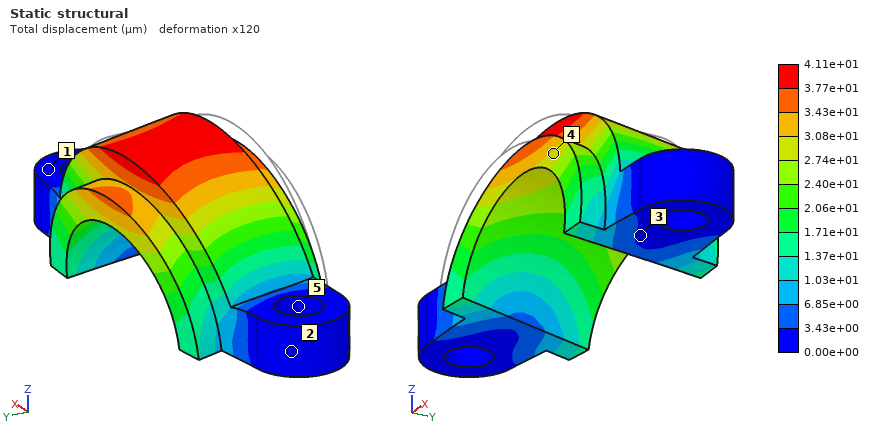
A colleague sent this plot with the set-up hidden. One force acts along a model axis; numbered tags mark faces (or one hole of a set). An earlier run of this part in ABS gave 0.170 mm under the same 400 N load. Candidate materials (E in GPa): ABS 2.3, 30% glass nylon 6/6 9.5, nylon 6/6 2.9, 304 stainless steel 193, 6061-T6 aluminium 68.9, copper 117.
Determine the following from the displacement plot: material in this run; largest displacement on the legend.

30% glass nylon 6/6
4.11e+01 µm
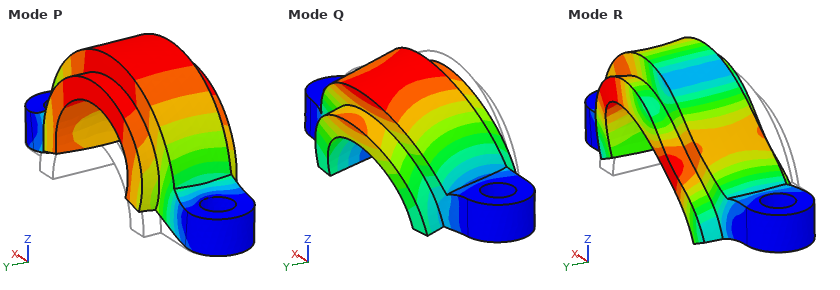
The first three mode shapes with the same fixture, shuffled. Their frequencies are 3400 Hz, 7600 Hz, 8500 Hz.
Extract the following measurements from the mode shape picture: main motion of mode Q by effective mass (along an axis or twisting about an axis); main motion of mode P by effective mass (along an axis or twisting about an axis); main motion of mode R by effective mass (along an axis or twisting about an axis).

along Y
along Z
along X
